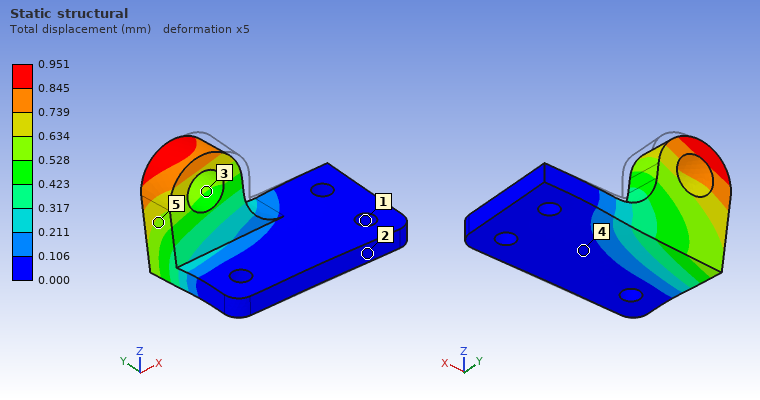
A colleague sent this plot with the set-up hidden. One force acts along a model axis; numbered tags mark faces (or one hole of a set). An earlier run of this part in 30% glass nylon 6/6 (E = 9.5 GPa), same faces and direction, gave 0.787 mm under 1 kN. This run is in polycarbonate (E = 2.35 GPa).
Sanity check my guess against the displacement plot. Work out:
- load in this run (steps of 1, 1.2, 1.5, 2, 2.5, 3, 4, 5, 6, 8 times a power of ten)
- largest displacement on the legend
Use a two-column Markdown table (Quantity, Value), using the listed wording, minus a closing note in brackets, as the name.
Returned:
| Quantity | Value |
|---|---|
| load in this run | 300 N |
| largest displacement on the legend | 0.951 mm |
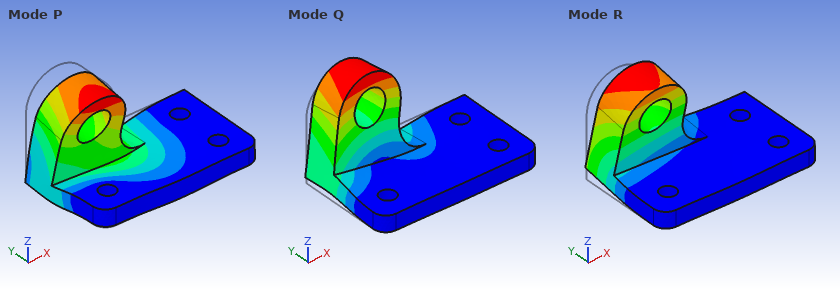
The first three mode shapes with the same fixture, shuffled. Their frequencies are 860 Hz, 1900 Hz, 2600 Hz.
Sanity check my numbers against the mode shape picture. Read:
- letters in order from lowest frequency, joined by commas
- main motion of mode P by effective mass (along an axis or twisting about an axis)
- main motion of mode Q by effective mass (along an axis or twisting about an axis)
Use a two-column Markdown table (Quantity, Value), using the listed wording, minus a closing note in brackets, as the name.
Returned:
| Quantity | Value |
|---|---|
| letters in order from lowest frequency, joined by commas | R, Q, P |
| main motion of mode P by effective mass | along Z |
| main motion of mode Q by effective mass | along X |
